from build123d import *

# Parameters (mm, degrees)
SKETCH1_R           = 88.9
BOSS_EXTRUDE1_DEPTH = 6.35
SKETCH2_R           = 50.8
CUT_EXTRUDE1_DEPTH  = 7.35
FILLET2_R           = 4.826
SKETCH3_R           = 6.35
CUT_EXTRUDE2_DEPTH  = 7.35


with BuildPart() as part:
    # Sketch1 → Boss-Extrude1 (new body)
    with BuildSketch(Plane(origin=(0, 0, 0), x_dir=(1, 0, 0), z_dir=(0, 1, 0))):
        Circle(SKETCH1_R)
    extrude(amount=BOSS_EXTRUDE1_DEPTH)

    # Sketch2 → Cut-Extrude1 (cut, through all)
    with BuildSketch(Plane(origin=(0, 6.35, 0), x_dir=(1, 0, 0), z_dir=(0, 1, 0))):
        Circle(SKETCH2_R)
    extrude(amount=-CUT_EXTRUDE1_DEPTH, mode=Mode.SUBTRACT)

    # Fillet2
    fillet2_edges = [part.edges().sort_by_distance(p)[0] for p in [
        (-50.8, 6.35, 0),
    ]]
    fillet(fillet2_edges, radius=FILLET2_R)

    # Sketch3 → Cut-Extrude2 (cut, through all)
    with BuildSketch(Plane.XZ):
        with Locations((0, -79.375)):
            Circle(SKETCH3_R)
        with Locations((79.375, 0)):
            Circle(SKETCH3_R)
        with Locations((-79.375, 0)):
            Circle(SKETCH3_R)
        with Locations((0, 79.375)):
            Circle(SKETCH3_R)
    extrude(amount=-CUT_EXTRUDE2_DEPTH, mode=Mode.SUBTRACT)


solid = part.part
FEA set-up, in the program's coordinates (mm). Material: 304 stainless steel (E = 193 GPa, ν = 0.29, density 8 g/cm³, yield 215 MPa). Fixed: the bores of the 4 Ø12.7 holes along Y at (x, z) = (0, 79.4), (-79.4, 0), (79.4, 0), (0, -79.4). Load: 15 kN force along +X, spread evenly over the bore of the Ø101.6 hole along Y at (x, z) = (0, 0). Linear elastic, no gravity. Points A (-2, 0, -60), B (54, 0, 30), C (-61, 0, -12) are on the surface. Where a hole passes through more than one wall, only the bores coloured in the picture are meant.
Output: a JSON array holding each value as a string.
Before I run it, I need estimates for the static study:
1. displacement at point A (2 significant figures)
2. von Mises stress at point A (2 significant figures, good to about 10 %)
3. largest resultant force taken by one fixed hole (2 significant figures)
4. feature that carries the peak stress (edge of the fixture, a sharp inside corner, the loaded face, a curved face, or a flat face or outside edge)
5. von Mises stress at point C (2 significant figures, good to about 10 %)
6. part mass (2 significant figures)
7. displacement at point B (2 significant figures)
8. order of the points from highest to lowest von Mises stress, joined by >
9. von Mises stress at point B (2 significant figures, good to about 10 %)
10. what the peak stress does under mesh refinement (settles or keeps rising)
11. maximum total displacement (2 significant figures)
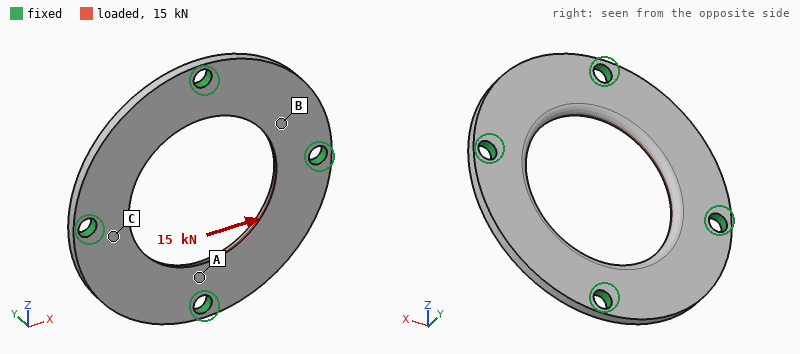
["3.2 µm", "6.1 MPa", "4.2 kN", "edge of the fixture", "27 MPa", "810 g", "5.4 µm", "C > B > A", "17 MPa", "keeps rising", "11 µm"]
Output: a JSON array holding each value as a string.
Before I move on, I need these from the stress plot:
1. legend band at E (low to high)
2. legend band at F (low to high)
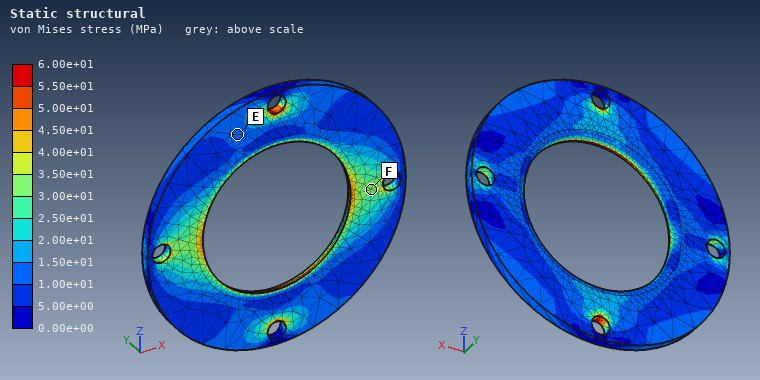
["1.00e+01 to 1.50e+01 MPa", "3.00e+01 to 3.50e+01 MPa"]
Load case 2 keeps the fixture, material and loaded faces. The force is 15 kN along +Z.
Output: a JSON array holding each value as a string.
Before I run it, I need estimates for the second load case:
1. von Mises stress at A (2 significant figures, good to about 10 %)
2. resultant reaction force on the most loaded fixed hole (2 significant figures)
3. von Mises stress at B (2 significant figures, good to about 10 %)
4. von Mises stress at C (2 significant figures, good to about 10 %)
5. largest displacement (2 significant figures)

["31 MPa", "4.2 kN", "9.8 MPa", "11 MPa", "11 µm"]
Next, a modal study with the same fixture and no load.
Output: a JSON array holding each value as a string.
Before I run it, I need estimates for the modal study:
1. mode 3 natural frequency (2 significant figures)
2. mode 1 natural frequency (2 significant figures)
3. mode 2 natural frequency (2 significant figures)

["2400 Hz", "2300 Hz", "2400 Hz"]
